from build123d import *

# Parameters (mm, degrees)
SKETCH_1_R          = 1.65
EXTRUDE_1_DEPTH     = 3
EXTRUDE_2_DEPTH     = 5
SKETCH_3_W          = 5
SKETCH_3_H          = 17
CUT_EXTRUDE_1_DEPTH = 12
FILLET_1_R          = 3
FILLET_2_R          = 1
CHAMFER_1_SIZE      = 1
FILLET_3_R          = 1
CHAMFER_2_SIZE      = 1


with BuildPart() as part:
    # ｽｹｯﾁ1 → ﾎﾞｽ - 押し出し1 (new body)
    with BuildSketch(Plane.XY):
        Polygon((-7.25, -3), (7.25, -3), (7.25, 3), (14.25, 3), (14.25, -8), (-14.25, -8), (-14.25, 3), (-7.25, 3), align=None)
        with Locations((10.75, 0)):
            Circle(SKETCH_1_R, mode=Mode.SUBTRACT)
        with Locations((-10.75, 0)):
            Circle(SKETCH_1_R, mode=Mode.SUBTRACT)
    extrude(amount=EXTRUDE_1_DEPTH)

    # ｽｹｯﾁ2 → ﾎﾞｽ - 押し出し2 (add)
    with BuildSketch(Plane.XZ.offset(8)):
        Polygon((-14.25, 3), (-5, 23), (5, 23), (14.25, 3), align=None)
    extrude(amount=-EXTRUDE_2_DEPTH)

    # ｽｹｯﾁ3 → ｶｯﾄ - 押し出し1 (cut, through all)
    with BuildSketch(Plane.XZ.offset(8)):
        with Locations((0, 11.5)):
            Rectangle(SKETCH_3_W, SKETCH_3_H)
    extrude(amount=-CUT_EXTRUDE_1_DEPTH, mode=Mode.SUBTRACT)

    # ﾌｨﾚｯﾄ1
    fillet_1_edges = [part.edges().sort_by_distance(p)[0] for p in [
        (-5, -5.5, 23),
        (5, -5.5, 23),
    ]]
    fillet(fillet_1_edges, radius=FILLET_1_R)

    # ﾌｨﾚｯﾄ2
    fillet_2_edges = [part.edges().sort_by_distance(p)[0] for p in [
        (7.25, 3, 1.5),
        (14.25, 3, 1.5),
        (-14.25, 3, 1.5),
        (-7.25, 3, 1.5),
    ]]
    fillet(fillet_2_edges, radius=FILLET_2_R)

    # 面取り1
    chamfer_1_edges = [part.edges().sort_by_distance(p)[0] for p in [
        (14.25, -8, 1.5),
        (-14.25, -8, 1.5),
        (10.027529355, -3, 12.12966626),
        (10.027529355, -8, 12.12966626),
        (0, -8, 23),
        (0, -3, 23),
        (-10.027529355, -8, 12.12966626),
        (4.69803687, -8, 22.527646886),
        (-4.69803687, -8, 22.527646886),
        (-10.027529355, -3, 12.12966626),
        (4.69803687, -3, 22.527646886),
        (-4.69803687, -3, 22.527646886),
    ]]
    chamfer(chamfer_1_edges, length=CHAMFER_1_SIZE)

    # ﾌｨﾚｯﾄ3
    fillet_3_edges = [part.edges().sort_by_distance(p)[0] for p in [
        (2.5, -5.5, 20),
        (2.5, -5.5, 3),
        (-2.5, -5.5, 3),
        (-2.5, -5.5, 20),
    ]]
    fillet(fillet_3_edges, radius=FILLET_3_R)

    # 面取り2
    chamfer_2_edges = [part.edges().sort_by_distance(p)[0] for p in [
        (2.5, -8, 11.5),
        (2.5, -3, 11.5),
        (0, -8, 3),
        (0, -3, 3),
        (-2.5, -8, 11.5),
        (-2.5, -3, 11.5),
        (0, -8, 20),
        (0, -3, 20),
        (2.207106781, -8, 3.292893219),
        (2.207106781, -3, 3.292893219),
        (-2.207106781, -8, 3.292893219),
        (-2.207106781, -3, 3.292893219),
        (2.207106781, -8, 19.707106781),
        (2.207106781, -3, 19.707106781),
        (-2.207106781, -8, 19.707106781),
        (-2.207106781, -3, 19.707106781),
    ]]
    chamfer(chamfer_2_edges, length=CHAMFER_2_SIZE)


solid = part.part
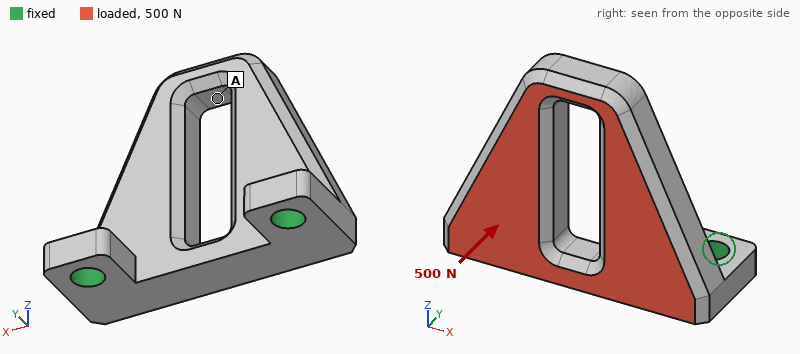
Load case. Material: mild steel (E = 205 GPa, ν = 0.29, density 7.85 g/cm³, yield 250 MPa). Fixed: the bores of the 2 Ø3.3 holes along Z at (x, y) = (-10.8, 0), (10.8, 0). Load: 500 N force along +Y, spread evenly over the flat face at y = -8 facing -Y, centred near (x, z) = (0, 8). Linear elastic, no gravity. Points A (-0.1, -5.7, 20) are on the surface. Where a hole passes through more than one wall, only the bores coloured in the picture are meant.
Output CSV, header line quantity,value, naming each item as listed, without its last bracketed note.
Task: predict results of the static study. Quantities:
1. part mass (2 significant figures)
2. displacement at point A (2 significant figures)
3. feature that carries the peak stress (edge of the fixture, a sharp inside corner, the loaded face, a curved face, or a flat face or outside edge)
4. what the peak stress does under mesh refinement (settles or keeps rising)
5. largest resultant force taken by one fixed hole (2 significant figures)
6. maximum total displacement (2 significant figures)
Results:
quantity,value
part mass,16 g
displacement at point A,40 µm
feature that carries the peak stress,edge of the fixture
what the peak stress does under mesh refinement,keeps rising
largest resultant force taken by one fixed hole,270 N
maximum total displacement,47 µm
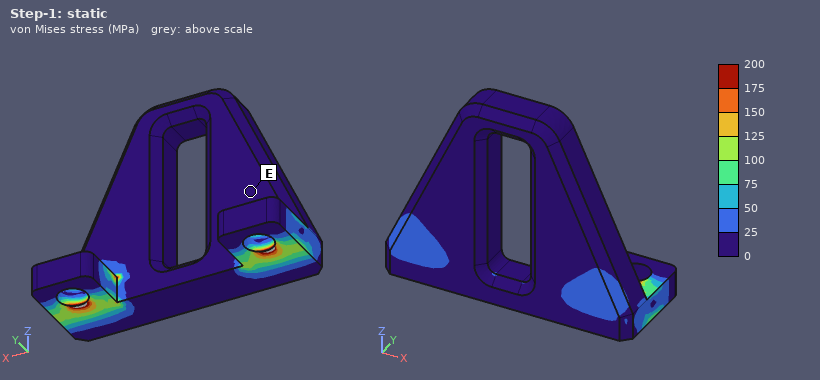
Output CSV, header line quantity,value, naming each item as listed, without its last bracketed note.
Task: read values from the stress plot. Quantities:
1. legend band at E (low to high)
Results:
quantity,value
legend band at E,0 to 25 MPa
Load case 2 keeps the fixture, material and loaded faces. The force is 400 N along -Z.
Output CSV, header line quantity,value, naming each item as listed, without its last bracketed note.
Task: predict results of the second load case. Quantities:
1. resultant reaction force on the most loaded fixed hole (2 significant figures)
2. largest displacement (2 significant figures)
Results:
quantity,value
resultant reaction force on the most loaded fixed hole,200 N
largest displacement,28 µm
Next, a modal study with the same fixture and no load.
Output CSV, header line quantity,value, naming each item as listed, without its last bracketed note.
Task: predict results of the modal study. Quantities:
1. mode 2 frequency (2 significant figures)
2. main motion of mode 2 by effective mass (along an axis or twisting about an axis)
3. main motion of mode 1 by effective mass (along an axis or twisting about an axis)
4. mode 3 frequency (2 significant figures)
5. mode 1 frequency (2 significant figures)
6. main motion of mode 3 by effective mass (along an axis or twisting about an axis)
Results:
quantity,value
mode 2 frequency,15 kHz
main motion of mode 2 by effective mass,along X
main motion of mode 1 by effective mass,along Y
mode 3 frequency,20 kHz
mode 1 frequency,5100 Hz
main motion of mode 3 by effective mass,along X
